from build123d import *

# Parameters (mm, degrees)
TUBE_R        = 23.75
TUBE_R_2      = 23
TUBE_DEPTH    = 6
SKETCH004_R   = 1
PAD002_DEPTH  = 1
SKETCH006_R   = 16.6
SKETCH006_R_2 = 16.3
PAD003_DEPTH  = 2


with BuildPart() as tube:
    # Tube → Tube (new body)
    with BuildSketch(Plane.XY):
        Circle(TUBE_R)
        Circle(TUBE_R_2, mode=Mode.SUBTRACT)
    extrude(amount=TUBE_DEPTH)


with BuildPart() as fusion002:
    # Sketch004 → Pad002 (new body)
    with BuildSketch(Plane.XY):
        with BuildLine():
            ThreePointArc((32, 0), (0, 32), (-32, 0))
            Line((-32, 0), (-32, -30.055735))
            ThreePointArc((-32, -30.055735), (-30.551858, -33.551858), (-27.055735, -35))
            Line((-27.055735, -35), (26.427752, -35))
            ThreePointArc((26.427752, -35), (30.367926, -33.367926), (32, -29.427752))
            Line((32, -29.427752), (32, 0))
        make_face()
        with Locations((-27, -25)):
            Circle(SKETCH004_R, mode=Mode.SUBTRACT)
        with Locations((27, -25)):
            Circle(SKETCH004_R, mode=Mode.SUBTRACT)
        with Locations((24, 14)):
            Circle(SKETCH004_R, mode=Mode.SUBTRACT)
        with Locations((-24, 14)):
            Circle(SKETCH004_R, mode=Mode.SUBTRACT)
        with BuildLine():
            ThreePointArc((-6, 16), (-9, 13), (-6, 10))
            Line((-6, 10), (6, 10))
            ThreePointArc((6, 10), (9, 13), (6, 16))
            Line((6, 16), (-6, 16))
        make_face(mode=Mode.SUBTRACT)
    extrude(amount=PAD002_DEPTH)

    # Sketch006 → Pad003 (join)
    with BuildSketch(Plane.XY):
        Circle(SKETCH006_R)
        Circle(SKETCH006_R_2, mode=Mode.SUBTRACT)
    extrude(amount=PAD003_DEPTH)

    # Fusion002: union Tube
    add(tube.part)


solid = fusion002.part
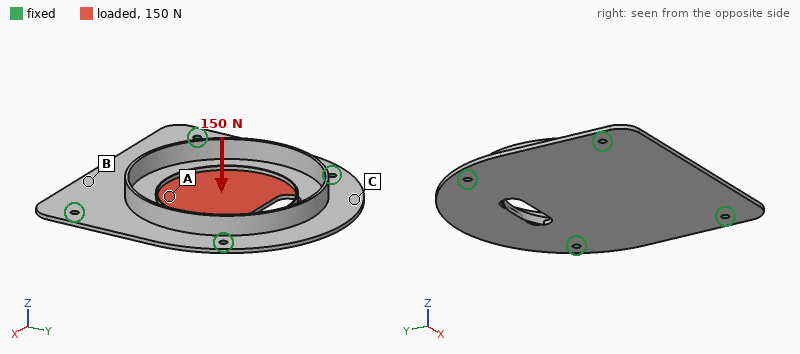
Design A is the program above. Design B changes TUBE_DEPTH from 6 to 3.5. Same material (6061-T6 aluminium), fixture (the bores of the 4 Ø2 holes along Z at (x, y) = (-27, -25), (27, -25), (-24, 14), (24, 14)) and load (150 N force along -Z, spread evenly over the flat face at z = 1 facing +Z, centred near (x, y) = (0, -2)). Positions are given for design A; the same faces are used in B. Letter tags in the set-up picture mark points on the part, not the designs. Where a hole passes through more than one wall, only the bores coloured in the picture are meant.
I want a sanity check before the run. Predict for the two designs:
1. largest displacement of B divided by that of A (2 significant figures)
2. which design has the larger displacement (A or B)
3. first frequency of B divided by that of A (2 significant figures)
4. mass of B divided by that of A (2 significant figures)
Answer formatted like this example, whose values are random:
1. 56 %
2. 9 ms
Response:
1. 1.3
2. B
3. 0.95
4. 0.94
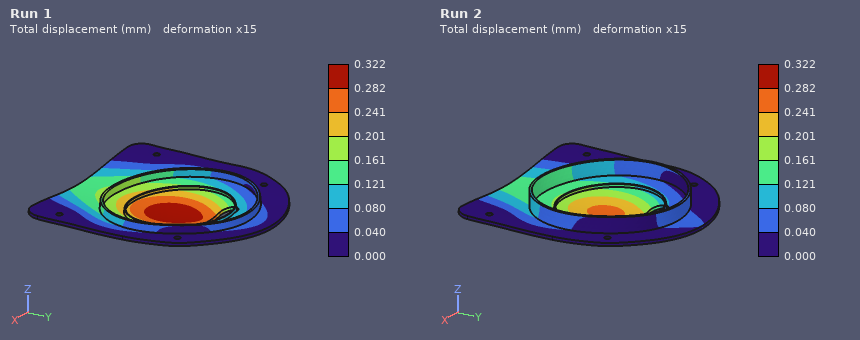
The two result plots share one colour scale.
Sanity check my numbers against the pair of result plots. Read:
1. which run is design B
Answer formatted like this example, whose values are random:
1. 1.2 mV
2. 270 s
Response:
1. Run 1
